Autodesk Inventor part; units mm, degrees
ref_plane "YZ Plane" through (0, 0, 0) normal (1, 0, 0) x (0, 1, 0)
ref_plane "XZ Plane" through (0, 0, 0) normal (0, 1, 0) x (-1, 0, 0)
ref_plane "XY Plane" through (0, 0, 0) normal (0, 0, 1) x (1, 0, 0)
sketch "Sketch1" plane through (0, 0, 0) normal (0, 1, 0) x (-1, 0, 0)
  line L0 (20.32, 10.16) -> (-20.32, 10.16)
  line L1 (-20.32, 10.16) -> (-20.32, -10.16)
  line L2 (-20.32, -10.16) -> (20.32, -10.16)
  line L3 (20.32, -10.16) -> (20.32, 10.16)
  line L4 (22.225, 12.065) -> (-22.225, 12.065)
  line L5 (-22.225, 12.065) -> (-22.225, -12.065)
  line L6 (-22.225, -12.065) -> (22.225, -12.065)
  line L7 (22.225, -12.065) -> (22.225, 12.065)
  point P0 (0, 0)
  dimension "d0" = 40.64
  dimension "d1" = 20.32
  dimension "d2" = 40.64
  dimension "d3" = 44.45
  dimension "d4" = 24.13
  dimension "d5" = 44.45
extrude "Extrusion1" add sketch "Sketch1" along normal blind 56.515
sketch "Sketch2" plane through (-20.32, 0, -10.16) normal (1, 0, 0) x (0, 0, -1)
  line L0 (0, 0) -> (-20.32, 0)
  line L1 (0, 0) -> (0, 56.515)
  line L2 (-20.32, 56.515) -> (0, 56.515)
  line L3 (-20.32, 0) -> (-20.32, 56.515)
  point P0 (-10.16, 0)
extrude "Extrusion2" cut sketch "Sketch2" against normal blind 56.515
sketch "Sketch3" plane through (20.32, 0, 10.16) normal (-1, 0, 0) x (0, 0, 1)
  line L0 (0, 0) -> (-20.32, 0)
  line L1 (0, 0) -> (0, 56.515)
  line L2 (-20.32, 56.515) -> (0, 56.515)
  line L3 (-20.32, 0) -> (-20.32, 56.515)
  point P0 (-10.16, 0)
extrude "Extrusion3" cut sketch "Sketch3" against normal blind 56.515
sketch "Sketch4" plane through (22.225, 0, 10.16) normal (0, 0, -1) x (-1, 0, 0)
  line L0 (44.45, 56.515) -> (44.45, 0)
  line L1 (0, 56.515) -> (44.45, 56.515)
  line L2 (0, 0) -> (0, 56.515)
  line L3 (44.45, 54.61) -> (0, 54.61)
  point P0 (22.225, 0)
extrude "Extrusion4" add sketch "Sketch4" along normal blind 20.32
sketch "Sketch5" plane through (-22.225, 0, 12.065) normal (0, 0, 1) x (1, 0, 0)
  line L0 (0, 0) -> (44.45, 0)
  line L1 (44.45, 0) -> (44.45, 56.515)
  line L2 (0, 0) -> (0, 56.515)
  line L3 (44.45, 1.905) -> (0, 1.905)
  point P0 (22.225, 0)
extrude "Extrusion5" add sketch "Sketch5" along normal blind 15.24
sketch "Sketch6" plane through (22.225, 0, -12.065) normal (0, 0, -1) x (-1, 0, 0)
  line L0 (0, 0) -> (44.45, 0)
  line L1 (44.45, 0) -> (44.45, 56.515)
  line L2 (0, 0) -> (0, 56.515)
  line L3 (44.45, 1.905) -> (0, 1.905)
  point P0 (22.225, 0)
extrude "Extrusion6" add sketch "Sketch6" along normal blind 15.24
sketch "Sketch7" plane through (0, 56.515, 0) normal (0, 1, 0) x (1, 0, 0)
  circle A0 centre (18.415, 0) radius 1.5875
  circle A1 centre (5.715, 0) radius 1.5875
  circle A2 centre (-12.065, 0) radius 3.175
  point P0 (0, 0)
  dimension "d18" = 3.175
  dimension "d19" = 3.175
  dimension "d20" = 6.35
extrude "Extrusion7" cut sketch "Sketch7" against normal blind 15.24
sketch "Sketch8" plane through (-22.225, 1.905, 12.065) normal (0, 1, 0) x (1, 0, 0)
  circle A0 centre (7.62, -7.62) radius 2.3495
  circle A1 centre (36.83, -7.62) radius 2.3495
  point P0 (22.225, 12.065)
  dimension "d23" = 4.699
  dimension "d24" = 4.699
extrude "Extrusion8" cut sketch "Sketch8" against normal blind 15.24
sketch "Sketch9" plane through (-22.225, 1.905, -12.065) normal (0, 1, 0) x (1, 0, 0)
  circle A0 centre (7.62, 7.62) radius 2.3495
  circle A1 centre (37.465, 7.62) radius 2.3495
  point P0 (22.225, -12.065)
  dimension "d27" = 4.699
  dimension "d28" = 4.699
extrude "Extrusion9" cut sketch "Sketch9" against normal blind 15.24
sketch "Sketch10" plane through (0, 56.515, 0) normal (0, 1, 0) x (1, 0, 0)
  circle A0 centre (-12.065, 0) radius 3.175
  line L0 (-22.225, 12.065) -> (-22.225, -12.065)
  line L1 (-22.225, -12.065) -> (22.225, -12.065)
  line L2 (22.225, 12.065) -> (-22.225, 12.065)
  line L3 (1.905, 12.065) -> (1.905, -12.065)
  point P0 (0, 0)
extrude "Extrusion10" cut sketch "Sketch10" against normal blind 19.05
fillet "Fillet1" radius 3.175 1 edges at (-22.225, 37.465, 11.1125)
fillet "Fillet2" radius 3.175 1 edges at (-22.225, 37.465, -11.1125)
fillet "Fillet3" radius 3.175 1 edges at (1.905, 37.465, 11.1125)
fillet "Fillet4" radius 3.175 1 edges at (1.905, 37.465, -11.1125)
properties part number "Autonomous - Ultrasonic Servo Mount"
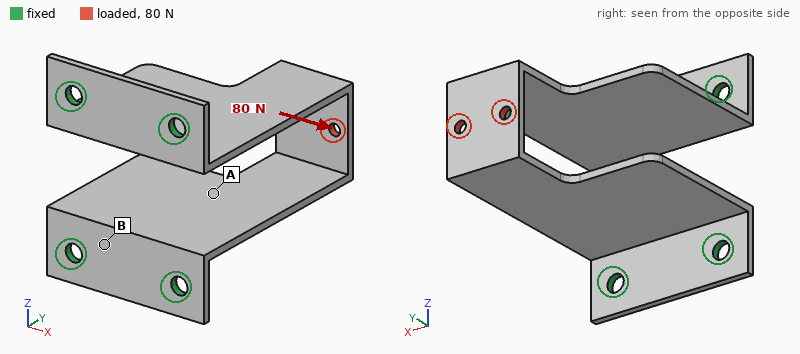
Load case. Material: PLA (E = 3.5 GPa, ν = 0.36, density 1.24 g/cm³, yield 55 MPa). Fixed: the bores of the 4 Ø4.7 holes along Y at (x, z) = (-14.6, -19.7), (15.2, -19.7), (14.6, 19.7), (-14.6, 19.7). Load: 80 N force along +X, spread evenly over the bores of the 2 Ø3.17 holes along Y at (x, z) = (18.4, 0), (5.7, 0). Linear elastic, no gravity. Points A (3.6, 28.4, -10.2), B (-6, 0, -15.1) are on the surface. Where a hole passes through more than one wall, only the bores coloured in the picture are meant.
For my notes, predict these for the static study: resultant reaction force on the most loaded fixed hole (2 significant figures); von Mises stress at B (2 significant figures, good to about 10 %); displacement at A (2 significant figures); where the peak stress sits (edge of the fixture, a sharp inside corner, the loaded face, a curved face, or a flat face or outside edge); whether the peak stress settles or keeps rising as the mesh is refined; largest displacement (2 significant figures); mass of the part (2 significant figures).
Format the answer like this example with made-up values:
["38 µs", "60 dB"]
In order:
["75 N", "7.3 MPa", "0.35 mm", "edge of the fixture", "keeps rising", "0.87 mm", "14 g"]
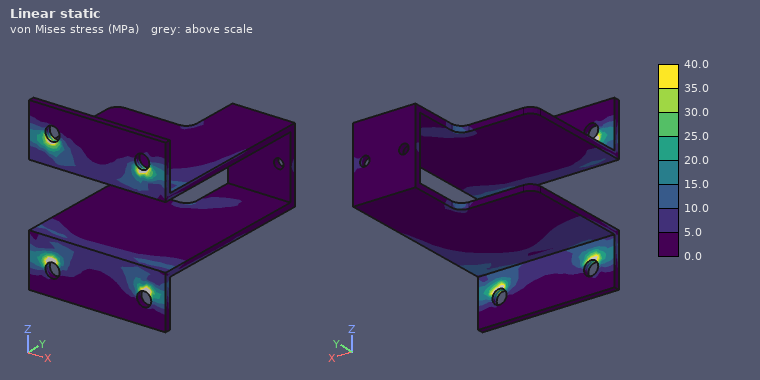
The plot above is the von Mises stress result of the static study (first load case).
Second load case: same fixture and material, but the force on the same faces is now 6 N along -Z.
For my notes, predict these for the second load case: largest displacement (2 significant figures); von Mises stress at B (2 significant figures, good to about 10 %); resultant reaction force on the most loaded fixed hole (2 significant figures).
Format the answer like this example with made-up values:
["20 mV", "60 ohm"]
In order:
["0.86 mm", "1.9 MPa", "4.5 N"]
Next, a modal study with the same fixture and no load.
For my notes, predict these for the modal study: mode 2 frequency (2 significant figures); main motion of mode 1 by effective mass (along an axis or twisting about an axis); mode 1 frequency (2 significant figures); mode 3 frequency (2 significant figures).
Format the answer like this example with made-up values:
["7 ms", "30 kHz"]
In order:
["600 Hz", "along Z", "230 Hz", "610 Hz"]
